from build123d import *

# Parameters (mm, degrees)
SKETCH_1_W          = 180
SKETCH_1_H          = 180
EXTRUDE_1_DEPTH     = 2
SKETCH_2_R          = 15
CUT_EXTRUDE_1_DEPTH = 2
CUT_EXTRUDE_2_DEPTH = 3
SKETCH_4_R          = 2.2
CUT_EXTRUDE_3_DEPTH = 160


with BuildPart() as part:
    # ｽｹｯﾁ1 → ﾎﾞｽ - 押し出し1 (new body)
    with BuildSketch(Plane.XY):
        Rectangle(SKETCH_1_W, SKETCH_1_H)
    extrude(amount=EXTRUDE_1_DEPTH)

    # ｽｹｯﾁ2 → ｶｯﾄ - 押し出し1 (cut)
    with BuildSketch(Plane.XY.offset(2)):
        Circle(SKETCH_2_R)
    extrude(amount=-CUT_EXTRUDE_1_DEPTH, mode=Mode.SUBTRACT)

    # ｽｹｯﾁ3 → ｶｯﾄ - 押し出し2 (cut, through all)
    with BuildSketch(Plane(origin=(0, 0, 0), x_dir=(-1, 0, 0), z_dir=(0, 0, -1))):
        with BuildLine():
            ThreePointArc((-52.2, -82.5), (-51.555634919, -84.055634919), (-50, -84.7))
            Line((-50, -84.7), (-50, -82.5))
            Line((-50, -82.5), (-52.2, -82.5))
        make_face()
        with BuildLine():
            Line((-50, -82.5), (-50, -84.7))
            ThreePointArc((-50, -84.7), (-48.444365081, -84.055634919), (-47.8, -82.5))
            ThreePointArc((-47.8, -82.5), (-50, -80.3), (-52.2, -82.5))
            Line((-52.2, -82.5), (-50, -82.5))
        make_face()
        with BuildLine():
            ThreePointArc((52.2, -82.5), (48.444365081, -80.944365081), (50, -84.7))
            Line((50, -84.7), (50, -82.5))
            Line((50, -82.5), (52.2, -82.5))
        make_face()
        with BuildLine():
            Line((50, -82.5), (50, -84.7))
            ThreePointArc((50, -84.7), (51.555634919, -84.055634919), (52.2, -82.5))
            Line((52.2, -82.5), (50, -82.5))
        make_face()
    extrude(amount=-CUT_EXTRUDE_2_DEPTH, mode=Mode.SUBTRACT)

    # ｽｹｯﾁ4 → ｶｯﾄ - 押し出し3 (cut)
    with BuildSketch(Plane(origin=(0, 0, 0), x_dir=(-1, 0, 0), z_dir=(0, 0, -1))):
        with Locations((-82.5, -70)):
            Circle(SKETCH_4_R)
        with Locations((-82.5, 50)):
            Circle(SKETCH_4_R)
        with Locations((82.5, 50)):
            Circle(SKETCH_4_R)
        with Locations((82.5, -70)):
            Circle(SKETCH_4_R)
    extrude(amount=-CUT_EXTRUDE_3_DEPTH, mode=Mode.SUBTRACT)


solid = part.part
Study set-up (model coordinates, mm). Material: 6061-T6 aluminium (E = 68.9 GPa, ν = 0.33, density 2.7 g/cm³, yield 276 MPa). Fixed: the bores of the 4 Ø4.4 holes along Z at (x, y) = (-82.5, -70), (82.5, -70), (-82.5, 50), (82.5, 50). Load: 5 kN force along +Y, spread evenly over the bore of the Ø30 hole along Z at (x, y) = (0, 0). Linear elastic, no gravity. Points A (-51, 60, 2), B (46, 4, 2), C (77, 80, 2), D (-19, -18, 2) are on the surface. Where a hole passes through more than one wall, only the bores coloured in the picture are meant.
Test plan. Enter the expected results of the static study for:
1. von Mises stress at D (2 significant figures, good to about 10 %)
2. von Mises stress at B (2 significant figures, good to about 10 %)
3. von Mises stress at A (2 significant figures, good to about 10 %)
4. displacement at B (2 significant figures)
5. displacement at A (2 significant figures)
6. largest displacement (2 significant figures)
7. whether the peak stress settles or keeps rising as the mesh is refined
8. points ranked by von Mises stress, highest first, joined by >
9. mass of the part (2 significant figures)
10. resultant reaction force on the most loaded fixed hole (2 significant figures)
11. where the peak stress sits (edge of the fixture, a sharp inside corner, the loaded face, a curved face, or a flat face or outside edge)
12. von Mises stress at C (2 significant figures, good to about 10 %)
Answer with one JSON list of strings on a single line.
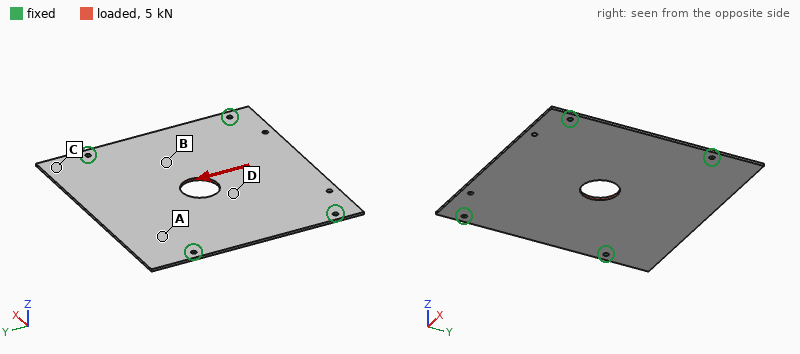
["21 MPa", "16 MPa", "10.0 MPa", "21 µm", "19 µm", "41 µm", "keeps rising", "D > B > A > C", "170 g", "1.4 kN", "edge of the fixture", "4.3 MPa"]
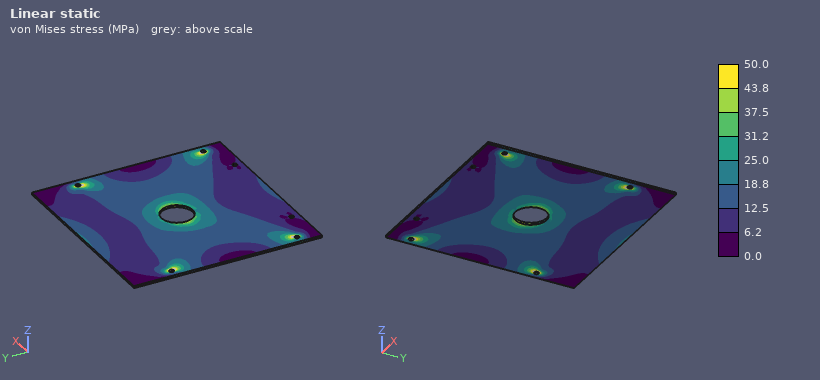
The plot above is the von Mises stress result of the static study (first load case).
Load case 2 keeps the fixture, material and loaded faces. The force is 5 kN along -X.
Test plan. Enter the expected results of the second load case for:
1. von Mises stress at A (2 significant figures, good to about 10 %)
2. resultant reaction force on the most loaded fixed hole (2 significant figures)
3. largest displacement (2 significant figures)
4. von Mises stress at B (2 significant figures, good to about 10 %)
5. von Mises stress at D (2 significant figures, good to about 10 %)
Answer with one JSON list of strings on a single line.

["9.8 MPa", "1.5 kN", "31 µm", "12 MPa", "19 MPa"]
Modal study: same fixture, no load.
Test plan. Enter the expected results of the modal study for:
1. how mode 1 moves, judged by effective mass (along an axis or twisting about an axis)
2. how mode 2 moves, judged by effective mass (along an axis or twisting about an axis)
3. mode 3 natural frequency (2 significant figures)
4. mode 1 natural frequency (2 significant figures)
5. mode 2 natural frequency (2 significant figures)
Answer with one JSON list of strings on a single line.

["along Z", "twisting about X", "530 Hz", "300 Hz", "370 Hz"]
